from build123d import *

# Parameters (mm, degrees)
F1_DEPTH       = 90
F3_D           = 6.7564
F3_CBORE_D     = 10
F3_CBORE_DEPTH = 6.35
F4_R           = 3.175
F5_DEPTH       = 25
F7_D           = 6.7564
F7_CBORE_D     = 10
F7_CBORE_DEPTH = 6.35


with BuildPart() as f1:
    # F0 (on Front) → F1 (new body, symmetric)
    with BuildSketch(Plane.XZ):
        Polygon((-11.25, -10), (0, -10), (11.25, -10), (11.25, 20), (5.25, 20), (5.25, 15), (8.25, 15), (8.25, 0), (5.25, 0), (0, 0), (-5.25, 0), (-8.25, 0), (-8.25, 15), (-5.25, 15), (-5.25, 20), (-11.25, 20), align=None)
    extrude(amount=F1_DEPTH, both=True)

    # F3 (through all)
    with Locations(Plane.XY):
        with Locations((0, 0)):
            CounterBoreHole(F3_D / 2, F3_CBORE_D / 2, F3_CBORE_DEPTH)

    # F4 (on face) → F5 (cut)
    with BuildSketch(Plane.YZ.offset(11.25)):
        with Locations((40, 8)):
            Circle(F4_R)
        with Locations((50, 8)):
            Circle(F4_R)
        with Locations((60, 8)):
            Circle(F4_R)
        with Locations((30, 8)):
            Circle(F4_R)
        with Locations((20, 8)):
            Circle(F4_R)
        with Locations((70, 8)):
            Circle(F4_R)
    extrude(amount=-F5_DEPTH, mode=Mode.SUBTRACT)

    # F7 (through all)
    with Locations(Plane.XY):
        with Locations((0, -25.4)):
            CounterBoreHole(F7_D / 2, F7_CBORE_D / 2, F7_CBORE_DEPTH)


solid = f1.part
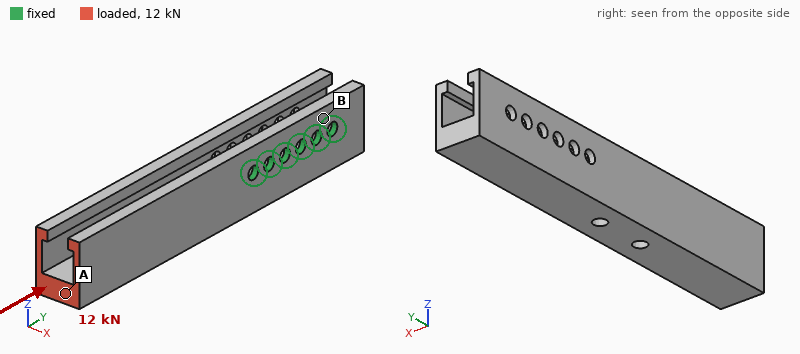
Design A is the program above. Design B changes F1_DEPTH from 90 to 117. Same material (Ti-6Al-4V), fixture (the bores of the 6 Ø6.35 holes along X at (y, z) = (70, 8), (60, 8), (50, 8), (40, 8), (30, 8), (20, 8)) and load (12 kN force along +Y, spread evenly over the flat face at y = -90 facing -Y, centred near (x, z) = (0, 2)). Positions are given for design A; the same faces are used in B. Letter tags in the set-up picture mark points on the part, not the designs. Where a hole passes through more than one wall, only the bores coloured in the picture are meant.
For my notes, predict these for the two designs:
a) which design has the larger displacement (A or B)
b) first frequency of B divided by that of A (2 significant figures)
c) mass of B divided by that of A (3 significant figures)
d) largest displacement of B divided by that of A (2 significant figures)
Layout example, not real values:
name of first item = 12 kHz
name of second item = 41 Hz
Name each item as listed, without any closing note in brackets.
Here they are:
which design has the larger displacement = B
first frequency of B divided by that of A = 0.74
mass of B divided by that of A = 1.31
largest displacement of B divided by that of A = 1.1
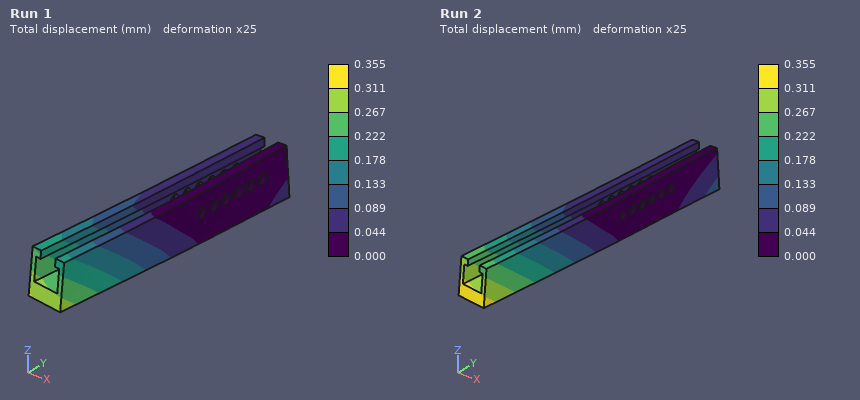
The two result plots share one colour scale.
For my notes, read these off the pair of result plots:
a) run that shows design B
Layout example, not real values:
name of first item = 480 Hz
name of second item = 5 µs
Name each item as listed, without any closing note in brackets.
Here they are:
run that shows design B = Run 2
